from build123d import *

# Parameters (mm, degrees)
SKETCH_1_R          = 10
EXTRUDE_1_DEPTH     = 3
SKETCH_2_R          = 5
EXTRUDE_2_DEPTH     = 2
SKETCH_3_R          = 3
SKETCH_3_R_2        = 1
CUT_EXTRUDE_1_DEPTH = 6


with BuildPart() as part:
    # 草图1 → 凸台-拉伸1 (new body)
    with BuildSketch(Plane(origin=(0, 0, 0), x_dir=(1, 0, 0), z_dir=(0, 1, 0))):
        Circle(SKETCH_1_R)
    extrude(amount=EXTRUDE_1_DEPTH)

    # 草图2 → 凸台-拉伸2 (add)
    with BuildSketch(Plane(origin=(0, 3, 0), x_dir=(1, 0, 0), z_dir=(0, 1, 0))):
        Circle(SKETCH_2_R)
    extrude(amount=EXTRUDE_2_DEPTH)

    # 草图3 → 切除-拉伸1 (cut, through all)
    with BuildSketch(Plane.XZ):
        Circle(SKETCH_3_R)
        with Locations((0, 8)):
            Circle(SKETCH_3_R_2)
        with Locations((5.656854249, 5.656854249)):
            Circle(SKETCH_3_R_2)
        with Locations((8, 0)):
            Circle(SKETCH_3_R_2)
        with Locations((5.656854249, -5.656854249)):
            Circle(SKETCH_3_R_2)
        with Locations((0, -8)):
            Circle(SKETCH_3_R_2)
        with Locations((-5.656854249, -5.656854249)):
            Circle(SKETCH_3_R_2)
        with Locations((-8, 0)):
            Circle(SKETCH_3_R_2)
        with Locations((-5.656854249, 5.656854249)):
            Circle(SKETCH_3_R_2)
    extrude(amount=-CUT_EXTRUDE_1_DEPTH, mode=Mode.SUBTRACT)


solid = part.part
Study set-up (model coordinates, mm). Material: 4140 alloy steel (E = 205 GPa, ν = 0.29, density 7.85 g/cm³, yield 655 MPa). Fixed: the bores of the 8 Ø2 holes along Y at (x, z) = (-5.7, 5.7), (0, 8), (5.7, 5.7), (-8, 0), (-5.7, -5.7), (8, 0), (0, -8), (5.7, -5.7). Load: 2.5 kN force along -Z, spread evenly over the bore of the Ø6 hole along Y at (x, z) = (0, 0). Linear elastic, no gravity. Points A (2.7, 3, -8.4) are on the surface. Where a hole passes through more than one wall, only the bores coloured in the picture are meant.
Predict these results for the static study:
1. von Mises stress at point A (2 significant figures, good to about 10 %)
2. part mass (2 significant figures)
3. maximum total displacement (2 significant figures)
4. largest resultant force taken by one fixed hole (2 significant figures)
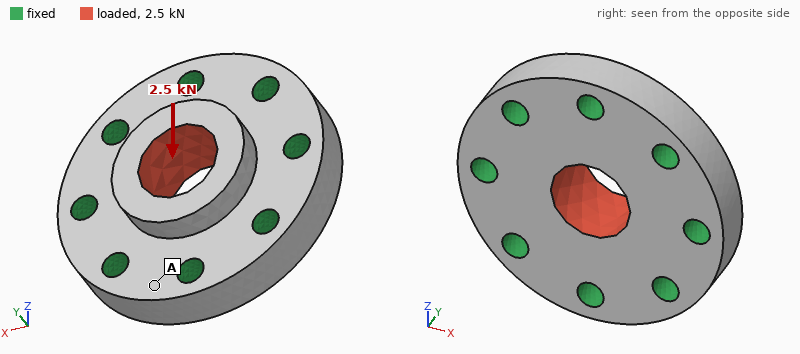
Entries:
8.2 MPa
6.9 g
1.9 µm
500 N
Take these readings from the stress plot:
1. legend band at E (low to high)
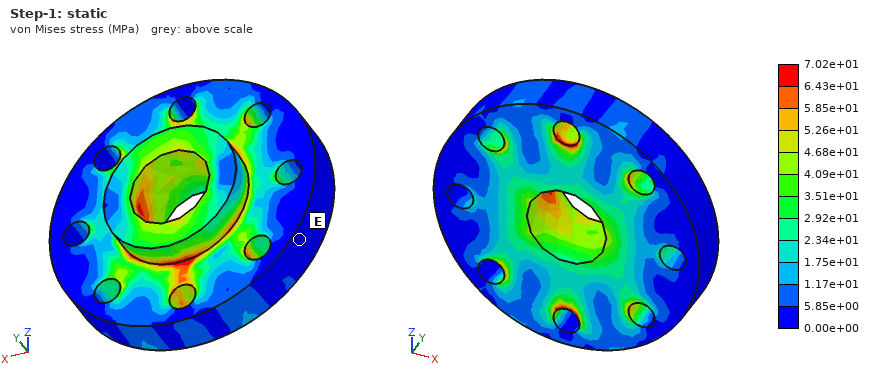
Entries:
0.00e+00 to 5.85e+00 MPa
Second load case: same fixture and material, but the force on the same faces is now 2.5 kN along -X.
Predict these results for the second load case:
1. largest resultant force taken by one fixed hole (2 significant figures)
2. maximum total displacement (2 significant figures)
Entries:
510 N
2.0 µm
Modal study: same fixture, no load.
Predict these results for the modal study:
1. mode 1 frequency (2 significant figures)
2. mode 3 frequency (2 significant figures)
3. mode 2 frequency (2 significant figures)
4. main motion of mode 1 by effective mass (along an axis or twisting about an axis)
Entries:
110 kHz
140 kHz
140 kHz
along Y
